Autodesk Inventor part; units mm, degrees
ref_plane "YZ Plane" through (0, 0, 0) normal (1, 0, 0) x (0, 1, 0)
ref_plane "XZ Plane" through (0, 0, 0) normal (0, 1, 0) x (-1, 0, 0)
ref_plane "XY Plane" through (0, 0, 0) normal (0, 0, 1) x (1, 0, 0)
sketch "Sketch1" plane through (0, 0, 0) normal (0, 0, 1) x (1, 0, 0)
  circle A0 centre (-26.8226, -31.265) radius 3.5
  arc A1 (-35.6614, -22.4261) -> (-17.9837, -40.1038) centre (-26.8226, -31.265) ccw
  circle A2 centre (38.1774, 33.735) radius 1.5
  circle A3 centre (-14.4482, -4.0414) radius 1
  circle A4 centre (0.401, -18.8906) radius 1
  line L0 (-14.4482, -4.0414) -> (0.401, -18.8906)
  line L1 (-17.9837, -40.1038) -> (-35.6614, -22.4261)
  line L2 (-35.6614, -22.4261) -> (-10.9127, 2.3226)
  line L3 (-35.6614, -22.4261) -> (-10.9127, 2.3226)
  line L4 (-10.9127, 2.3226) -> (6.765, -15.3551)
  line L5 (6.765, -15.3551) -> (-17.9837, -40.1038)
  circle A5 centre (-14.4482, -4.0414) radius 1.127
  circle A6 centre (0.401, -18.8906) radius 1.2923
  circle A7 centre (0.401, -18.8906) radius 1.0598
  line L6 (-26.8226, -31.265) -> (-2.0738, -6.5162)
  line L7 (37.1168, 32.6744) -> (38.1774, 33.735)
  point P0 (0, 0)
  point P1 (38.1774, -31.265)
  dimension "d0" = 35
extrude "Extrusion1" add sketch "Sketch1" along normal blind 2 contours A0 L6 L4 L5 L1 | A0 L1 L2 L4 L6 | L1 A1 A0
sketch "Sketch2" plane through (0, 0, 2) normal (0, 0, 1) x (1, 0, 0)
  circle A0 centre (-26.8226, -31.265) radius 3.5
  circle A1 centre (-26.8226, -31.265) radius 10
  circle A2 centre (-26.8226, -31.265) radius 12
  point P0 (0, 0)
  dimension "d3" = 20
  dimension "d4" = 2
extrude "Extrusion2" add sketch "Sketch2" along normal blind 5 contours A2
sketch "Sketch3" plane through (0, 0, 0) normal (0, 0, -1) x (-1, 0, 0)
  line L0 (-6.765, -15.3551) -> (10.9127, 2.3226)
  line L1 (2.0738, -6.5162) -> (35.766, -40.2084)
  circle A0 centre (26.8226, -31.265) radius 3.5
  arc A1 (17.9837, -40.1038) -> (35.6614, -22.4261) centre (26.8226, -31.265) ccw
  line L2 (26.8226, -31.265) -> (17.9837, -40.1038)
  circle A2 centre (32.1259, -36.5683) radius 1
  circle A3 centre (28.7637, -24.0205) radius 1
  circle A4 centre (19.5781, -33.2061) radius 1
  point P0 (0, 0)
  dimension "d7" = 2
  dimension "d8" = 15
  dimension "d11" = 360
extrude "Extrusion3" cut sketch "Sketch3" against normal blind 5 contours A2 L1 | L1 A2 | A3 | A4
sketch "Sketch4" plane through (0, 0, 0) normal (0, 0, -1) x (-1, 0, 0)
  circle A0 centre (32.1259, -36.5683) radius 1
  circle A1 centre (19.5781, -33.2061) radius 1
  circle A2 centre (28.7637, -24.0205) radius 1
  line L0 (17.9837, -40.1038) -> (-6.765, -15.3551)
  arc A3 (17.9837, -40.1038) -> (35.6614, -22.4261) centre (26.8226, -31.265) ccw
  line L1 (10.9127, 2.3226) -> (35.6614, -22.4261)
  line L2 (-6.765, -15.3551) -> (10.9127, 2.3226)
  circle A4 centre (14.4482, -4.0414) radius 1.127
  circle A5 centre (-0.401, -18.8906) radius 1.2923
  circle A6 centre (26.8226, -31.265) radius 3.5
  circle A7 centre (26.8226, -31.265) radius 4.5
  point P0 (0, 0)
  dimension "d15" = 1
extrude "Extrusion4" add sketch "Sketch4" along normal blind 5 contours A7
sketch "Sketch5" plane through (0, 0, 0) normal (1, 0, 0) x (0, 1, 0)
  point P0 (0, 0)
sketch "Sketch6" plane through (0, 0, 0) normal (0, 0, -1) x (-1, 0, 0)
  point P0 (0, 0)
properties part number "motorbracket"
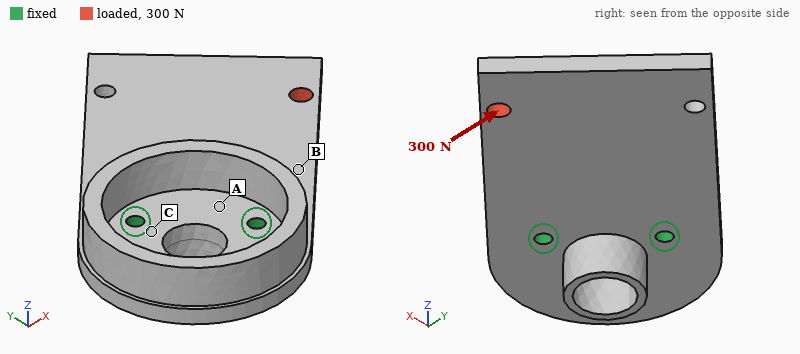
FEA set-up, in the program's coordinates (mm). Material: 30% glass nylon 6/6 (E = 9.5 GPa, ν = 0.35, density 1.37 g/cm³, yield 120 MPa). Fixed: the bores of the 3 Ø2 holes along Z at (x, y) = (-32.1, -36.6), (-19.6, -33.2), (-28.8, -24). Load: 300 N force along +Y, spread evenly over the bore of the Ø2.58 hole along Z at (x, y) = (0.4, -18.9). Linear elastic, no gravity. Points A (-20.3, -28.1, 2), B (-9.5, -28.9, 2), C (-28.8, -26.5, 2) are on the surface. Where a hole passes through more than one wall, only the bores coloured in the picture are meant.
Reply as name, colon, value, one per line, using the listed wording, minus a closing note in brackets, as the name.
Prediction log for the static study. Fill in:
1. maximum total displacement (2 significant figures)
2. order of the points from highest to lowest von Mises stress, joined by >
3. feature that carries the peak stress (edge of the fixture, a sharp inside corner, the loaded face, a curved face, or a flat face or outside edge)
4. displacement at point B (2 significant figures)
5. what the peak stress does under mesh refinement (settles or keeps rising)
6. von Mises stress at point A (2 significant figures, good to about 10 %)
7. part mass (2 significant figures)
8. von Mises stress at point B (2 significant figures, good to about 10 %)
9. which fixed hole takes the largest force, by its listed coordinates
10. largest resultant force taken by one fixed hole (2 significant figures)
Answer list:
maximum total displacement: 0.20 mm
order of the points from highest to lowest von Mises stress, joined by >: B > A > C
feature that carries the peak stress: edge of the fixture
displacement at point B: 0.063 mm
what the peak stress does under mesh refinement: keeps rising
von Mises stress at point A: 16 MPa
part mass: 4.0 g
von Mises stress at point B: 26 MPa
which fixed hole takes the largest force, by its listed coordinates: (-19.6, -33.2)
largest resultant force taken by one fixed hole: 550 N
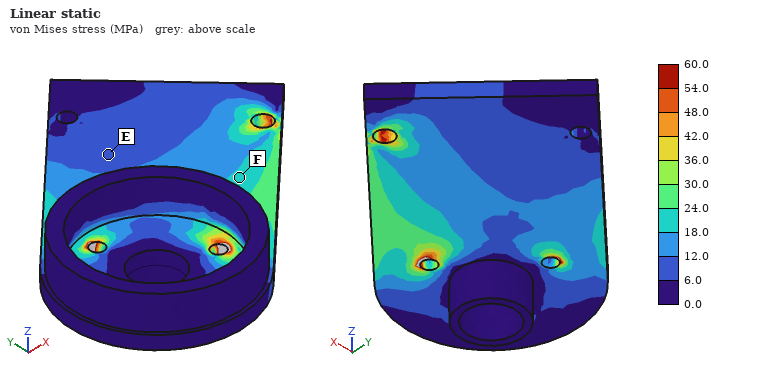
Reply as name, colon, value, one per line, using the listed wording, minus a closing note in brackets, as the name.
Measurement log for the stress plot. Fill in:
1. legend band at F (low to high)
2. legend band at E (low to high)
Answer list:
legend band at F: 18.0 to 24.0 MPa
legend band at E: 6.0 to 12.0 MPa
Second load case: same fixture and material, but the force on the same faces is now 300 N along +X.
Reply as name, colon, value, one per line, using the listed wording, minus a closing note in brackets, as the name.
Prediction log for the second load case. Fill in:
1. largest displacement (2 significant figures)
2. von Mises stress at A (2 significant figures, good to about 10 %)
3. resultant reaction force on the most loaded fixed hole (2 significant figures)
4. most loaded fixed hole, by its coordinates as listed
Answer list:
largest displacement: 77 µm
von Mises stress at A: 8.1 MPa
resultant reaction force on the most loaded fixed hole: 300 N
most loaded fixed hole, by its coordinates as listed: (-28.8, -24)
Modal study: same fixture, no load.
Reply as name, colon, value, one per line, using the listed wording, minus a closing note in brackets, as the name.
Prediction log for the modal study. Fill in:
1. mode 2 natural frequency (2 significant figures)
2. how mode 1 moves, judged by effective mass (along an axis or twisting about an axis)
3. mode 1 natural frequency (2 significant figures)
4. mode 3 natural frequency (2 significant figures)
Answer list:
mode 2 natural frequency: 2700 Hz
how mode 1 moves, judged by effective mass: along Z
mode 1 natural frequency: 1100 Hz
mode 3 natural frequency: 5700 Hz
